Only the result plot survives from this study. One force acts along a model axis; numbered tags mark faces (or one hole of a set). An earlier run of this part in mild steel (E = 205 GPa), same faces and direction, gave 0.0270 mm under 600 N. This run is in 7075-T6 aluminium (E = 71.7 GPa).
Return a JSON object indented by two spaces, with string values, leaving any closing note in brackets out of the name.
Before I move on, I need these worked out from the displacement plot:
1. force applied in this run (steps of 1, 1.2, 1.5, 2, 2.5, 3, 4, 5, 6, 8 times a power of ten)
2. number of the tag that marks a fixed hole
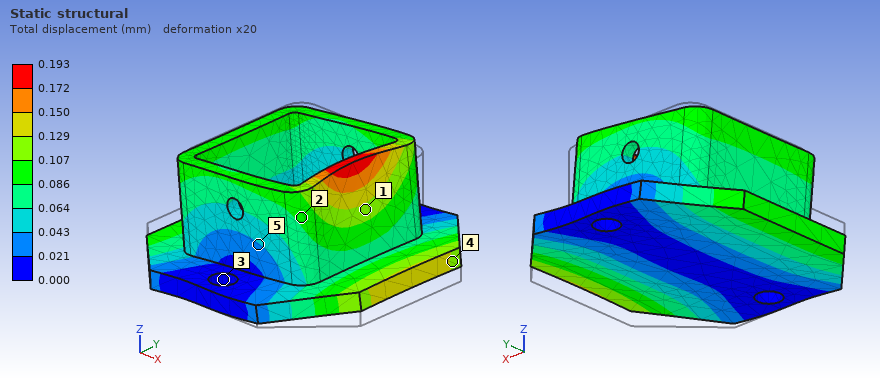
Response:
{
  "force applied in this run": "1.5 kN",
  "number of the tag that marks a fixed hole": "3"
}
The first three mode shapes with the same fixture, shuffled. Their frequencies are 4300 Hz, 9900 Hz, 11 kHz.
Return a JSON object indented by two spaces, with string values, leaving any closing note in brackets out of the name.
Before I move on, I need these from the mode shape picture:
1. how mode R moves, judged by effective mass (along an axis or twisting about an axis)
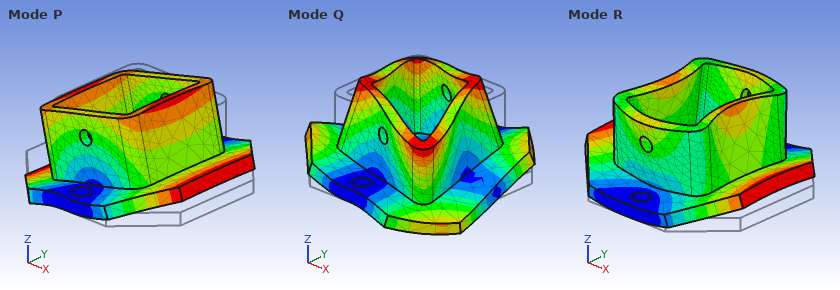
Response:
{
  "how mode R moves, judged by effective mass": "along Z"
}
